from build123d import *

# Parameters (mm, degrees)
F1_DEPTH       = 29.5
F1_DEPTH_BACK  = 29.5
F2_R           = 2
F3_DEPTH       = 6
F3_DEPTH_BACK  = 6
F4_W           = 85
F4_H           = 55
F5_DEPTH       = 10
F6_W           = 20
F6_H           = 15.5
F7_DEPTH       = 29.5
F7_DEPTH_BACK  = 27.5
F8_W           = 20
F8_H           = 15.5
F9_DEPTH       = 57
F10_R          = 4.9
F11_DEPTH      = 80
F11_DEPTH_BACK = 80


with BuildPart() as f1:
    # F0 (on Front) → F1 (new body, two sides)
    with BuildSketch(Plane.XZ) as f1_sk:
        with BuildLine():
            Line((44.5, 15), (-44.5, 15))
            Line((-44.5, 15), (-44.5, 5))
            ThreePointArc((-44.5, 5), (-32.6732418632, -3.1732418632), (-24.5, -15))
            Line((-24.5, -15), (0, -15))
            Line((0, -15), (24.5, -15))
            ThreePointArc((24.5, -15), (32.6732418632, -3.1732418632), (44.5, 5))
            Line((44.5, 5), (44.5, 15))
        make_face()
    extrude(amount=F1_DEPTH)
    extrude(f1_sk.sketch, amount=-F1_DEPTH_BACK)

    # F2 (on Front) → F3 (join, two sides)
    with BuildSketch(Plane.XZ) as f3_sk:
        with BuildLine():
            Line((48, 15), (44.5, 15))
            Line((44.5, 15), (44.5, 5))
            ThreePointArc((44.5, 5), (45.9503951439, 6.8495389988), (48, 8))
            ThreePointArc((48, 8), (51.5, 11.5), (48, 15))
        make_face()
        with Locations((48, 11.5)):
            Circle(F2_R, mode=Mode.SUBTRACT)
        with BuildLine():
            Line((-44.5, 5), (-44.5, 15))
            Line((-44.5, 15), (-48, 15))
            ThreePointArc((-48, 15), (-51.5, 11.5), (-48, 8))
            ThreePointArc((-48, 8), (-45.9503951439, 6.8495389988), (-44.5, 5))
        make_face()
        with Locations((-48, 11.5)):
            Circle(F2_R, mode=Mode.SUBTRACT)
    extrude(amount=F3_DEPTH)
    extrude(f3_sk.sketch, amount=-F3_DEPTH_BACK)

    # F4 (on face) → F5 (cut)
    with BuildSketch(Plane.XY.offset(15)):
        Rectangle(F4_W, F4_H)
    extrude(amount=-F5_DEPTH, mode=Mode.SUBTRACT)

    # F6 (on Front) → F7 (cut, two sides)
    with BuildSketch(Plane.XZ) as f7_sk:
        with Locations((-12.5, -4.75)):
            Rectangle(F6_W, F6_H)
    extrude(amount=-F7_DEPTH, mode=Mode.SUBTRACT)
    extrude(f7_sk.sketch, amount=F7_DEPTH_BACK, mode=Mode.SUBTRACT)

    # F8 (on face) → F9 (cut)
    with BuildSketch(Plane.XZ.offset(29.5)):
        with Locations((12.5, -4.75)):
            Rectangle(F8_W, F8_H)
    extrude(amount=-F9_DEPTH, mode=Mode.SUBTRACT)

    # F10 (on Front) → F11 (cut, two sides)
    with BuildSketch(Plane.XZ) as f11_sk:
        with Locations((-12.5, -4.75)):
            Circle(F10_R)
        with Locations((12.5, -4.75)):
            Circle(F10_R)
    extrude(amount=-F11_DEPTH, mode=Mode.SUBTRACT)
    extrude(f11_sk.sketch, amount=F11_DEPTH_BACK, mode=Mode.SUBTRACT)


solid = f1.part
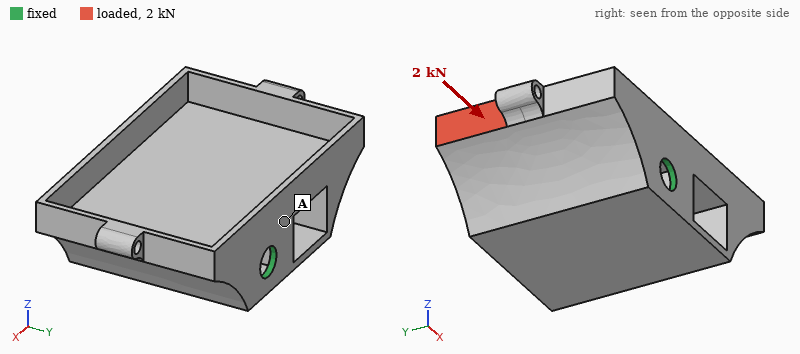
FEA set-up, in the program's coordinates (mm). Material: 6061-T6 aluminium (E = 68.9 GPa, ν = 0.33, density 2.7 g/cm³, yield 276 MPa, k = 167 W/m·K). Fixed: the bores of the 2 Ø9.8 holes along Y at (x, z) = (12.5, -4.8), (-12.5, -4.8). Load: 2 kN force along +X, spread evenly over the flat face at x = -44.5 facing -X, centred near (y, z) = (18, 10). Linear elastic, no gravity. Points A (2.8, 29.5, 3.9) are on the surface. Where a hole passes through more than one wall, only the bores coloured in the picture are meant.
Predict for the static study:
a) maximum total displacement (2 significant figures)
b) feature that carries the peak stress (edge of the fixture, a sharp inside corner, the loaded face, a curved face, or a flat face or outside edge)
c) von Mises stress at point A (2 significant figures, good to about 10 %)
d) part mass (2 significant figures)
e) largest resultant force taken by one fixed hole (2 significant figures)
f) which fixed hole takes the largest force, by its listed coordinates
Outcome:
0.37 mm
a curved face
35 MPa
130 g
1.6 kN
(12.5, -4.8)
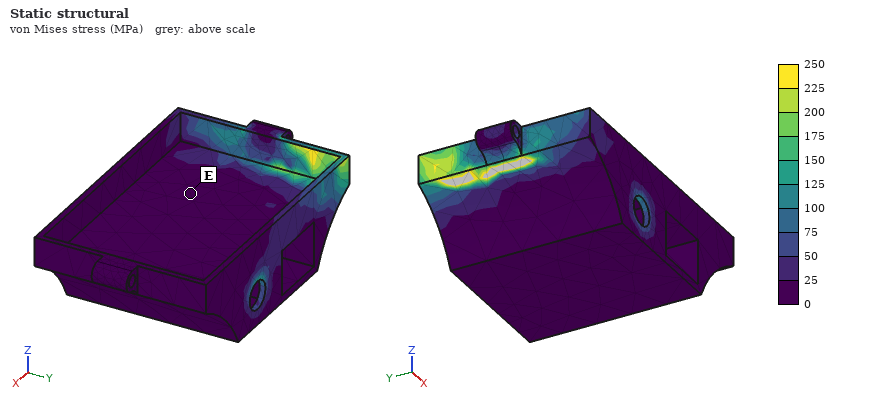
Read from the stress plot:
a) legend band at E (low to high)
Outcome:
0 to 25 MPa
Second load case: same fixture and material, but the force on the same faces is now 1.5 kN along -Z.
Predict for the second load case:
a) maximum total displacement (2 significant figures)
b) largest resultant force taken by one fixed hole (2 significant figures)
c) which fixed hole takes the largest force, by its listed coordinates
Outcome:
0.33 mm
1.0 kN
(12.5, -4.8)
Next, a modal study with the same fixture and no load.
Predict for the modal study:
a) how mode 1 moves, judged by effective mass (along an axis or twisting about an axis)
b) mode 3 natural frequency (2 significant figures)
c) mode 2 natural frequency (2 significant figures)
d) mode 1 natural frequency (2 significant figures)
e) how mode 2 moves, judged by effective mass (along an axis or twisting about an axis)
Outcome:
twisting about Y
5700 Hz
4100 Hz
2700 Hz
along Z
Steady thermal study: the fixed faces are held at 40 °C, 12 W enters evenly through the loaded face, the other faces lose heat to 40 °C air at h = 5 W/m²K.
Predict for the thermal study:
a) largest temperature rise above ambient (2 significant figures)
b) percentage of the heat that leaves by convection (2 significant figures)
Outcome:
22 K
5.0 %
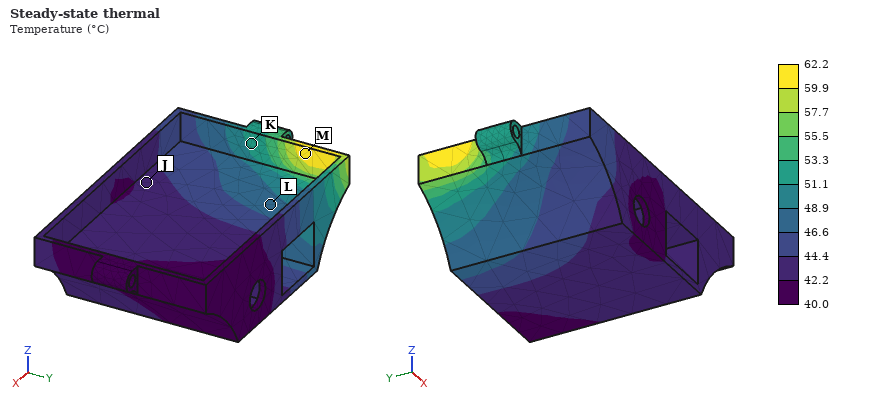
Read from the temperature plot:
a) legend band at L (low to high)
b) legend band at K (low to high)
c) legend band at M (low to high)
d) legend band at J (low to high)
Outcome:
46.6 to 48.9 °C
51.1 to 53.3 °C
59.9 to 62.2 °C
42.2 to 44.4 °C
